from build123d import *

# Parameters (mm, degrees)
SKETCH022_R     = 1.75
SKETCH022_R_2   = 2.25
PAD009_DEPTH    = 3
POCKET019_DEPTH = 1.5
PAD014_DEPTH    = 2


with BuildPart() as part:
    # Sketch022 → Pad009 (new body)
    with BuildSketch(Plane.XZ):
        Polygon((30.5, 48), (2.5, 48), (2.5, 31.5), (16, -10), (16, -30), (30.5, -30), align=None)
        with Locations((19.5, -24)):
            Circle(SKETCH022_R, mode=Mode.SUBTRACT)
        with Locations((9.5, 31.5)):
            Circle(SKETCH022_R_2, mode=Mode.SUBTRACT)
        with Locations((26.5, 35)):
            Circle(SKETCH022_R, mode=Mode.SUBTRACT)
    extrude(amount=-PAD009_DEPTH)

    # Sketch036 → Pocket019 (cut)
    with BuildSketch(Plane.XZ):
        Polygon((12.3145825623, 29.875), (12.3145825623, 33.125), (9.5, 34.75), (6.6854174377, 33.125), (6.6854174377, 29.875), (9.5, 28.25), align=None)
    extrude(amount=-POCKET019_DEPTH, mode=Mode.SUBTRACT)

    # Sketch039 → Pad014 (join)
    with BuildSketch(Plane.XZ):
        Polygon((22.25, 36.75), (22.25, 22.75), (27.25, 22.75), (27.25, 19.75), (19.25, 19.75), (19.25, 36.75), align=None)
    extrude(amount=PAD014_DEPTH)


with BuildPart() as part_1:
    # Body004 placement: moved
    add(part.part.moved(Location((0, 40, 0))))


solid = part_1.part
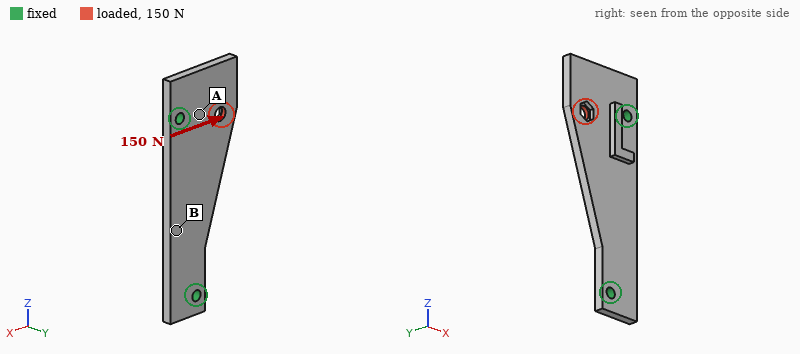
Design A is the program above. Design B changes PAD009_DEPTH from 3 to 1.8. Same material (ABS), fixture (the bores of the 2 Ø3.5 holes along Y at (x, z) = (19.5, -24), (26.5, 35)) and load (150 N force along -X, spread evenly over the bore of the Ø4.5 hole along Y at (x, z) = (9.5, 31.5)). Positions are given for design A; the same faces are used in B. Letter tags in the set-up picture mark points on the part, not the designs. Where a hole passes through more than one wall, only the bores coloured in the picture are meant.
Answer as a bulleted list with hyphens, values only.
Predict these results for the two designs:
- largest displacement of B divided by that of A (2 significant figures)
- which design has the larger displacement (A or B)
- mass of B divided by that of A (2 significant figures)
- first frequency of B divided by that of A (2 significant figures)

- 4.1
- B
- 0.61
- 0.64
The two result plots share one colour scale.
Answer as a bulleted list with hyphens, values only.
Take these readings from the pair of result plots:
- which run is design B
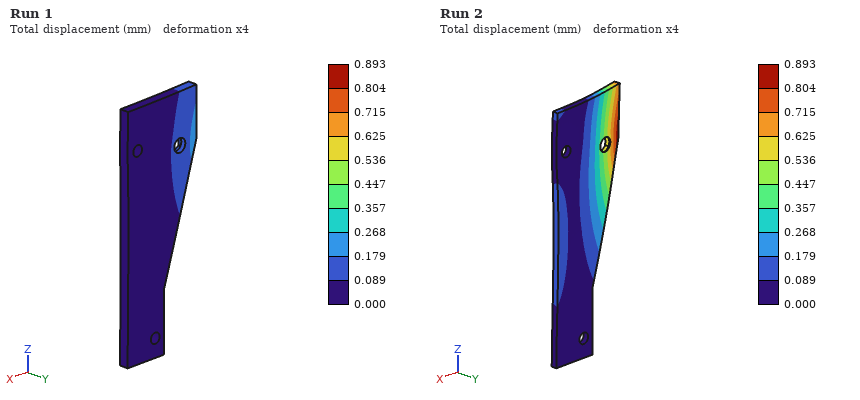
- Run 2
